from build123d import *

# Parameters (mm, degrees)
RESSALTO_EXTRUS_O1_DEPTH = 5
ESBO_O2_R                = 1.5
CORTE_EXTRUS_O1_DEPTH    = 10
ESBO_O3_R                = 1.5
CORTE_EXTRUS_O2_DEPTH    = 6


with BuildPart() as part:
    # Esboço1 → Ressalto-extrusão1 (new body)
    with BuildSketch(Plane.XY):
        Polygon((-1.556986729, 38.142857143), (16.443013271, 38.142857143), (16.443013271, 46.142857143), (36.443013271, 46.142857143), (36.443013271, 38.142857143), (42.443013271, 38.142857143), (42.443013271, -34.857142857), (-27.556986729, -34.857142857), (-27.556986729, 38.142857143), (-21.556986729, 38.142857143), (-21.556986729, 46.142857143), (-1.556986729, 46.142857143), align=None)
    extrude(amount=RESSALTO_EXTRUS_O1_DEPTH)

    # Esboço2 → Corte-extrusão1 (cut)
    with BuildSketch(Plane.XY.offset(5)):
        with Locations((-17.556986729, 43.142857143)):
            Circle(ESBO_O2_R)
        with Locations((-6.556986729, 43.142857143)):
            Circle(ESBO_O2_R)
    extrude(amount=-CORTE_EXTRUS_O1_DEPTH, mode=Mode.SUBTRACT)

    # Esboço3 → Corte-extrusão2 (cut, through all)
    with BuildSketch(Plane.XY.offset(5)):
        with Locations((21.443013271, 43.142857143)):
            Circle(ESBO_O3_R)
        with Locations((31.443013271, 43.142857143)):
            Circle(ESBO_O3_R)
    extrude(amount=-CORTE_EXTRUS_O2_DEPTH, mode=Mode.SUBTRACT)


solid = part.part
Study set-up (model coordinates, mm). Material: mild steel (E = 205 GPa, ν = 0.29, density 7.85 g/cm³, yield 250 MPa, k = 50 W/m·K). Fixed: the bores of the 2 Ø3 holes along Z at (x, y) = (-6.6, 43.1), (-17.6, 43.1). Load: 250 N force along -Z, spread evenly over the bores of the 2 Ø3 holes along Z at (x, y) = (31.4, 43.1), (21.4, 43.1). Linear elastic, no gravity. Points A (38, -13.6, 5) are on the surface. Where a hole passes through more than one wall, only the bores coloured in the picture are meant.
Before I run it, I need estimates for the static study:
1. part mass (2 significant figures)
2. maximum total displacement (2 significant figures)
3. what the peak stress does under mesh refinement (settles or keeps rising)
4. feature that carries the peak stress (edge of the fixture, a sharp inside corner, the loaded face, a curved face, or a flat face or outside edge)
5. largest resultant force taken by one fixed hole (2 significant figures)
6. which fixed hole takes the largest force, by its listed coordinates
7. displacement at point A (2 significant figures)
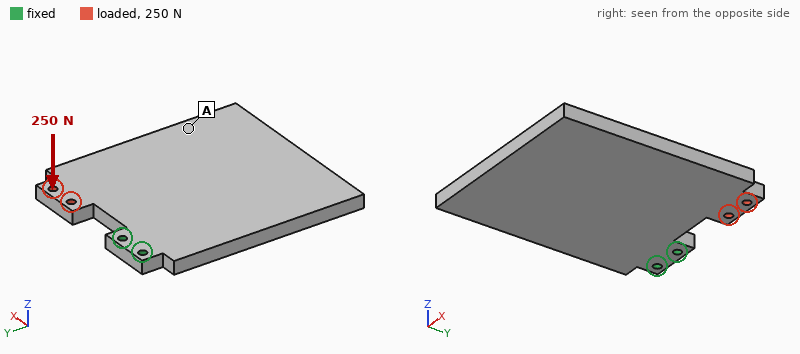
210 g
0.14 mm
keeps rising
edge of the fixture
690 N
(-6.6, 43.1)
0.058 mm
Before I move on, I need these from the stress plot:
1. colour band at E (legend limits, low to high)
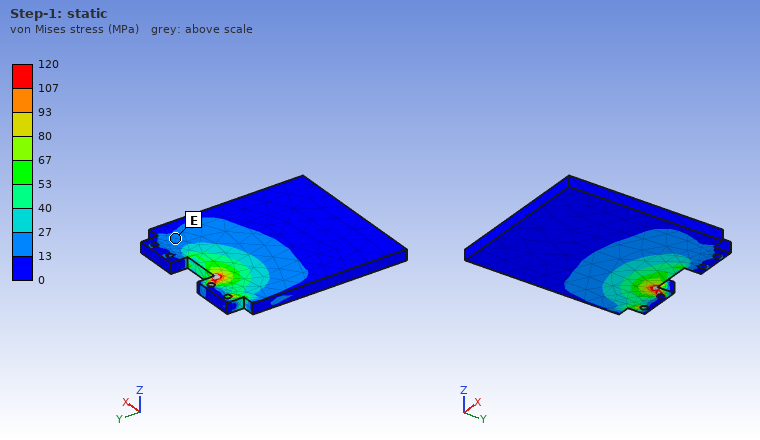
13 to 27 MPa
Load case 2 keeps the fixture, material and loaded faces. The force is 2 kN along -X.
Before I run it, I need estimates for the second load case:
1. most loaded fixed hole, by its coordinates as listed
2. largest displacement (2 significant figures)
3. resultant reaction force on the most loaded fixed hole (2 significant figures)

(-6.6, 43.1)
22 µm
1.2 kN
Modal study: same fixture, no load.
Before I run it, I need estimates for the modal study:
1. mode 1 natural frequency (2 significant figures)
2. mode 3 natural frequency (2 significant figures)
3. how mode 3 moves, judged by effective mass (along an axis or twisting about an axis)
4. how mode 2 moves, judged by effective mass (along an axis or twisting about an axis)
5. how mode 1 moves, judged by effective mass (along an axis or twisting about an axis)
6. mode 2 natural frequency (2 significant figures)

420 Hz
1500 Hz
along X
twisting about Y
along Z
960 Hz
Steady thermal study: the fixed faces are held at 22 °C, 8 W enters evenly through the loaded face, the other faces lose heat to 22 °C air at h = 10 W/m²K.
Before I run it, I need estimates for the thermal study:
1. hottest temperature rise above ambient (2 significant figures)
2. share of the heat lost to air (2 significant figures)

56 K
33 %
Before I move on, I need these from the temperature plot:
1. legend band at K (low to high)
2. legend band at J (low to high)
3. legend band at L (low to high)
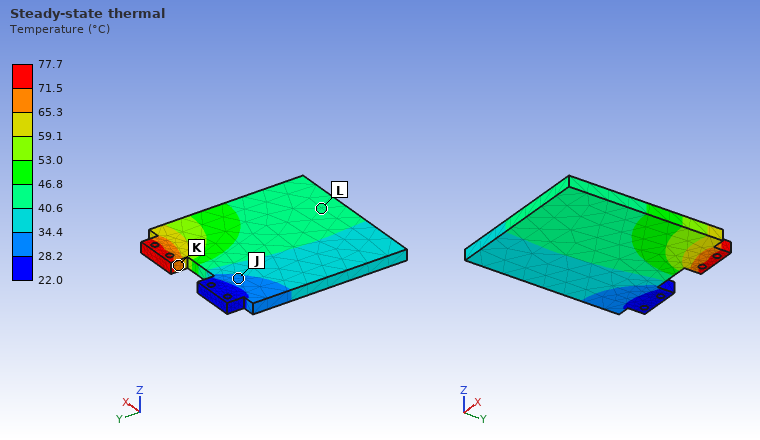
65.3 to 71.5 °C
28.2 to 34.4 °C
40.6 to 46.8 °C
